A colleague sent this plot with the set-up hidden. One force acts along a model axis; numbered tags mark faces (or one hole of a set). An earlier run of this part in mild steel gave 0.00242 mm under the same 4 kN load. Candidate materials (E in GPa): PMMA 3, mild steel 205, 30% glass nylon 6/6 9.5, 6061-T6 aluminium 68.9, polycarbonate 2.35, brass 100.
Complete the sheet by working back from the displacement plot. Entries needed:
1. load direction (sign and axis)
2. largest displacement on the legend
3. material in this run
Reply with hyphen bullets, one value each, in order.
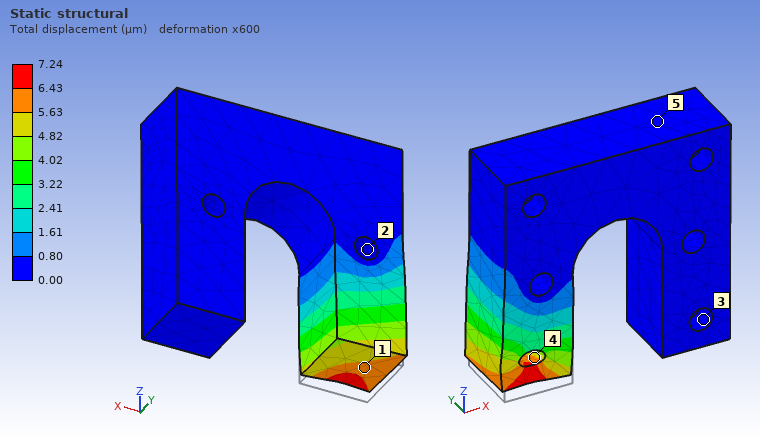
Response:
- +Z
- 7.24 µm
- 6061-T6 aluminium
